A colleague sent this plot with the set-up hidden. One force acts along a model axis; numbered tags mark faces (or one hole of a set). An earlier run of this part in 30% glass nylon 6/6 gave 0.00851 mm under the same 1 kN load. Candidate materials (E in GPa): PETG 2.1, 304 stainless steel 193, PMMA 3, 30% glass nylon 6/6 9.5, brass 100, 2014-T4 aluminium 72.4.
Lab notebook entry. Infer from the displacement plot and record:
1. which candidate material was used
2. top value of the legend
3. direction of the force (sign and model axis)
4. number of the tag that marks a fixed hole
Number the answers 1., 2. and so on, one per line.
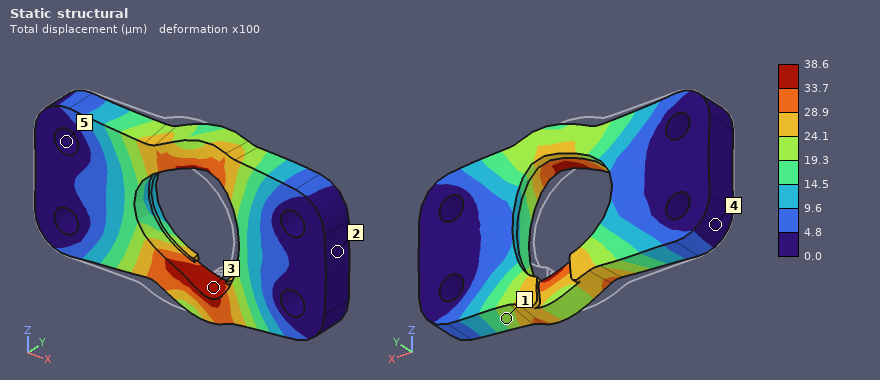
1. PETG
2. 38.6 µm
3. +X
4. 5
